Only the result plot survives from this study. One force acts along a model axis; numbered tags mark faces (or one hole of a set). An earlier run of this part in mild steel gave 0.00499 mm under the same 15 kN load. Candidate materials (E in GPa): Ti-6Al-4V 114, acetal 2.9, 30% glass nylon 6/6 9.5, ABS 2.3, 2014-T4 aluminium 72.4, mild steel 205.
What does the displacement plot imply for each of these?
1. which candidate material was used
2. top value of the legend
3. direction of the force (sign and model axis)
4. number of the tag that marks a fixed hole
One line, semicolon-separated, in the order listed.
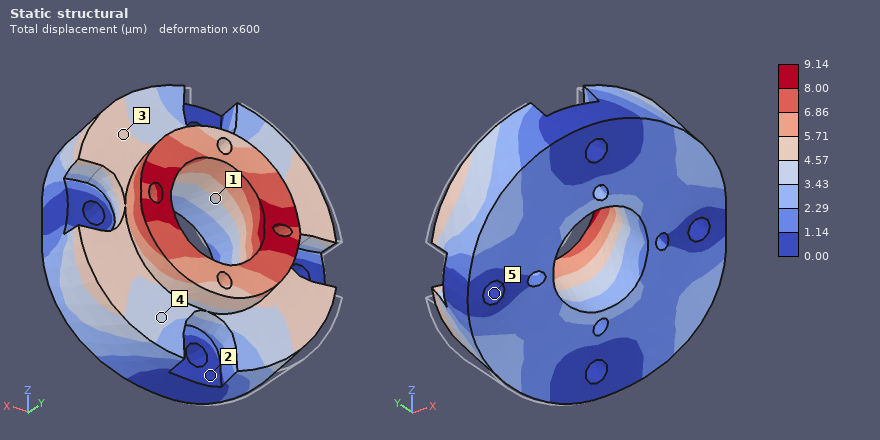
Ti-6Al-4V; 9.14 µm; +X; 5
